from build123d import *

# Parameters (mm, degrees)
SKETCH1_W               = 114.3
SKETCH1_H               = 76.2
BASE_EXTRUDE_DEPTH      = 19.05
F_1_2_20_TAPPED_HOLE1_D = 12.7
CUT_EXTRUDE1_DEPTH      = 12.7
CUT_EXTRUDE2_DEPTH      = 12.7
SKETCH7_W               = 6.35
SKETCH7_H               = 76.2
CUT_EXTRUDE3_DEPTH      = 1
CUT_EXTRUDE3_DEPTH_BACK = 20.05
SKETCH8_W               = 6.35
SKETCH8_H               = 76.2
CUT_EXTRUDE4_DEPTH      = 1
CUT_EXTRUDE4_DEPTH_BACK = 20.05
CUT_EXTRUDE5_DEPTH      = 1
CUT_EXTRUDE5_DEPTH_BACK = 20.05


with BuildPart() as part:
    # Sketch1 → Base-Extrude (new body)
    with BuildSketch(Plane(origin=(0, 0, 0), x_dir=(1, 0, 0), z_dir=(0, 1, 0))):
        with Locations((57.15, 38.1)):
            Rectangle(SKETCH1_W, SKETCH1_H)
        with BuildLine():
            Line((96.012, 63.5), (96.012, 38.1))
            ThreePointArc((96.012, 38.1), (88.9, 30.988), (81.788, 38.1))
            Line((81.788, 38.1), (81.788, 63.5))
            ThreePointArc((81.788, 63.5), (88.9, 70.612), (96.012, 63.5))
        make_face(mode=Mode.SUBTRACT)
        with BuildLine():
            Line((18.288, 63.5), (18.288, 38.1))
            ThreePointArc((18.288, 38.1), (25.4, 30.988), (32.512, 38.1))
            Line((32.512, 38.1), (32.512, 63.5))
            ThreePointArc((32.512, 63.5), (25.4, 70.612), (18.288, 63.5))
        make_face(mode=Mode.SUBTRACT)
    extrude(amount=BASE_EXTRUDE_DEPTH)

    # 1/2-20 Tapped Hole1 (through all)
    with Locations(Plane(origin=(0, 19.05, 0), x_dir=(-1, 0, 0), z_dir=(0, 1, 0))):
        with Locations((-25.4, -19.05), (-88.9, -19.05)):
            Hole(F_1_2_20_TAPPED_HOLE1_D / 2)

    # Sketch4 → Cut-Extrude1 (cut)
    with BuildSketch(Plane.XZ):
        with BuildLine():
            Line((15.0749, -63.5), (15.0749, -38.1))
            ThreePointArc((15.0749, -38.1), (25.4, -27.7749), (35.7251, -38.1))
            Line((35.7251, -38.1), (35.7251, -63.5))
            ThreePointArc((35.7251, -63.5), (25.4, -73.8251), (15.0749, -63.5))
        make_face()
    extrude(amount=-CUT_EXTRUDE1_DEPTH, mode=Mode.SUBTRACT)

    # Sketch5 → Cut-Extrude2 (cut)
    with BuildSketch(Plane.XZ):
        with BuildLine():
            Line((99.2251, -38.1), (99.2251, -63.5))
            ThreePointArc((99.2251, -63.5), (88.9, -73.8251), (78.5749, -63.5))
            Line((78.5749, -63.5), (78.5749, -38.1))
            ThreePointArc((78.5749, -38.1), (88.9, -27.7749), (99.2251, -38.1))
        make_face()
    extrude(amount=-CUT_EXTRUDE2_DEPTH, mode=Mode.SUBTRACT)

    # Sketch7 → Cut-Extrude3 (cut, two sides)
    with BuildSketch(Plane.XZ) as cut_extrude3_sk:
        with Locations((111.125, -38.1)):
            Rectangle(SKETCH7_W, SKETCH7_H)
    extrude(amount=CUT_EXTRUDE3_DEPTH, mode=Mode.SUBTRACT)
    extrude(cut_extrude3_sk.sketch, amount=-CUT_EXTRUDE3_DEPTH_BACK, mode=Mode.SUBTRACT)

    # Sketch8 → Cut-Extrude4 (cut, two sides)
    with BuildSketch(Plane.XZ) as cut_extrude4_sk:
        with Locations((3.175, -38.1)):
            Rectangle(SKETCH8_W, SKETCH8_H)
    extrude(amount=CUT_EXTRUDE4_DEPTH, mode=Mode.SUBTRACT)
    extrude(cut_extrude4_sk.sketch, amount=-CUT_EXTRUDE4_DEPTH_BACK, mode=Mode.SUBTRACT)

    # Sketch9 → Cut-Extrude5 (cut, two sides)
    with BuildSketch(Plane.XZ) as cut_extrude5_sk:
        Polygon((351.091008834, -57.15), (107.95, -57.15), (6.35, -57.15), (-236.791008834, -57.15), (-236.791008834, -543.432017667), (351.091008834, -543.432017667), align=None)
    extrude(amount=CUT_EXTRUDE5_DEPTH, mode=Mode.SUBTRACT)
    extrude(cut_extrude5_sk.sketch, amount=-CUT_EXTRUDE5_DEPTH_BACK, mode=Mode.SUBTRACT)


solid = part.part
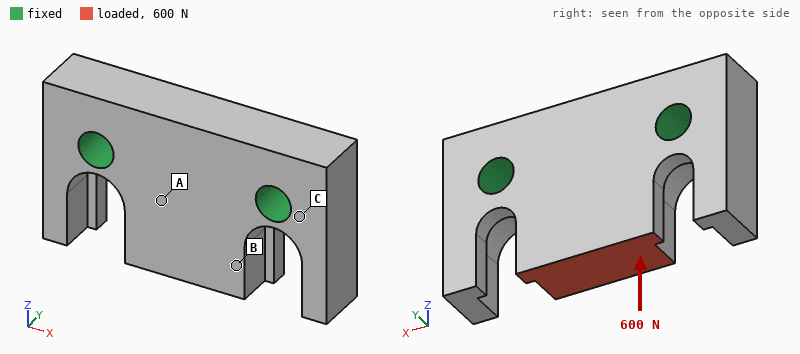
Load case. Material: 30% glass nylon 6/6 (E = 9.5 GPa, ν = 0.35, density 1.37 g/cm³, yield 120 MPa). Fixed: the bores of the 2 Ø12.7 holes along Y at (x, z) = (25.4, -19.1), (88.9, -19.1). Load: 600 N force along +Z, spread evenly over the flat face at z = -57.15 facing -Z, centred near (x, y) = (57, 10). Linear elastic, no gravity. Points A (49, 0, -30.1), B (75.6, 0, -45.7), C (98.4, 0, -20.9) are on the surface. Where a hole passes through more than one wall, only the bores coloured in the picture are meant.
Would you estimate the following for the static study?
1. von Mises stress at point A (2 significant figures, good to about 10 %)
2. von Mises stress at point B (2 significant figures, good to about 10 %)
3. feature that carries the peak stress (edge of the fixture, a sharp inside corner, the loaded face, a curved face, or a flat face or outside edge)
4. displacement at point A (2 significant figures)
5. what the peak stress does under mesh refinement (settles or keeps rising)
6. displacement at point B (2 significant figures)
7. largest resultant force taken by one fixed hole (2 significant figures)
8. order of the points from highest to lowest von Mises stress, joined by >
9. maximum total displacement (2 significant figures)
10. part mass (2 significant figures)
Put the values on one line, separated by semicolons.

0.44 MPa; 0.83 MPa; edge of the fixture; 2.8 µm; keeps rising; 3.5 µm; 310 N; B > A > C; 4.4 µm; 120 g
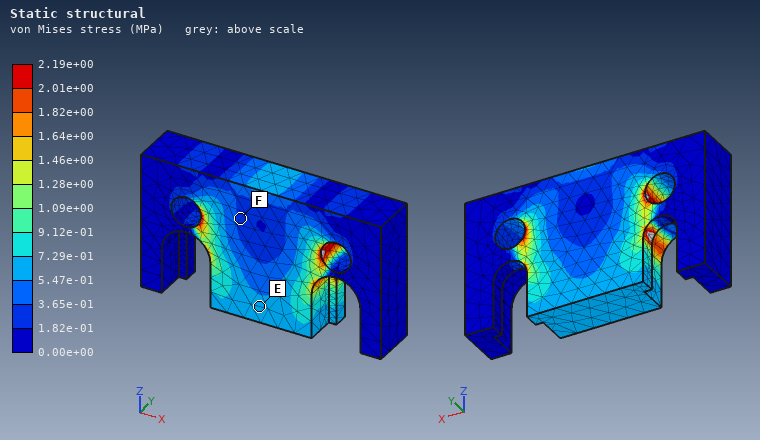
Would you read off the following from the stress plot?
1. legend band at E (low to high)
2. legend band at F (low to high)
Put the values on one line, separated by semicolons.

5.47e-01 to 7.29e-01 MPa; 1.82e-01 to 3.65e-01 MPa
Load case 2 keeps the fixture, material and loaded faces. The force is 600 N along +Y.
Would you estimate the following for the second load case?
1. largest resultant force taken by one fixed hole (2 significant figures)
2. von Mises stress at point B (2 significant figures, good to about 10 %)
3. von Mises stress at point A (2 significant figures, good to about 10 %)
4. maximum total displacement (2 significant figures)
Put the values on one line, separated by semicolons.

300 N; 2.8 MPa; 4.2 MPa; 76 µm
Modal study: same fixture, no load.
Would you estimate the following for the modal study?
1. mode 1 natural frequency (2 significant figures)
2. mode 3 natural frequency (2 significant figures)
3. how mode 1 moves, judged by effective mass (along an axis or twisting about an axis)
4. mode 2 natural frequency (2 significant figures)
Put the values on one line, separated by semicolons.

3900 Hz; 4400 Hz; along Y; 4400 Hz
